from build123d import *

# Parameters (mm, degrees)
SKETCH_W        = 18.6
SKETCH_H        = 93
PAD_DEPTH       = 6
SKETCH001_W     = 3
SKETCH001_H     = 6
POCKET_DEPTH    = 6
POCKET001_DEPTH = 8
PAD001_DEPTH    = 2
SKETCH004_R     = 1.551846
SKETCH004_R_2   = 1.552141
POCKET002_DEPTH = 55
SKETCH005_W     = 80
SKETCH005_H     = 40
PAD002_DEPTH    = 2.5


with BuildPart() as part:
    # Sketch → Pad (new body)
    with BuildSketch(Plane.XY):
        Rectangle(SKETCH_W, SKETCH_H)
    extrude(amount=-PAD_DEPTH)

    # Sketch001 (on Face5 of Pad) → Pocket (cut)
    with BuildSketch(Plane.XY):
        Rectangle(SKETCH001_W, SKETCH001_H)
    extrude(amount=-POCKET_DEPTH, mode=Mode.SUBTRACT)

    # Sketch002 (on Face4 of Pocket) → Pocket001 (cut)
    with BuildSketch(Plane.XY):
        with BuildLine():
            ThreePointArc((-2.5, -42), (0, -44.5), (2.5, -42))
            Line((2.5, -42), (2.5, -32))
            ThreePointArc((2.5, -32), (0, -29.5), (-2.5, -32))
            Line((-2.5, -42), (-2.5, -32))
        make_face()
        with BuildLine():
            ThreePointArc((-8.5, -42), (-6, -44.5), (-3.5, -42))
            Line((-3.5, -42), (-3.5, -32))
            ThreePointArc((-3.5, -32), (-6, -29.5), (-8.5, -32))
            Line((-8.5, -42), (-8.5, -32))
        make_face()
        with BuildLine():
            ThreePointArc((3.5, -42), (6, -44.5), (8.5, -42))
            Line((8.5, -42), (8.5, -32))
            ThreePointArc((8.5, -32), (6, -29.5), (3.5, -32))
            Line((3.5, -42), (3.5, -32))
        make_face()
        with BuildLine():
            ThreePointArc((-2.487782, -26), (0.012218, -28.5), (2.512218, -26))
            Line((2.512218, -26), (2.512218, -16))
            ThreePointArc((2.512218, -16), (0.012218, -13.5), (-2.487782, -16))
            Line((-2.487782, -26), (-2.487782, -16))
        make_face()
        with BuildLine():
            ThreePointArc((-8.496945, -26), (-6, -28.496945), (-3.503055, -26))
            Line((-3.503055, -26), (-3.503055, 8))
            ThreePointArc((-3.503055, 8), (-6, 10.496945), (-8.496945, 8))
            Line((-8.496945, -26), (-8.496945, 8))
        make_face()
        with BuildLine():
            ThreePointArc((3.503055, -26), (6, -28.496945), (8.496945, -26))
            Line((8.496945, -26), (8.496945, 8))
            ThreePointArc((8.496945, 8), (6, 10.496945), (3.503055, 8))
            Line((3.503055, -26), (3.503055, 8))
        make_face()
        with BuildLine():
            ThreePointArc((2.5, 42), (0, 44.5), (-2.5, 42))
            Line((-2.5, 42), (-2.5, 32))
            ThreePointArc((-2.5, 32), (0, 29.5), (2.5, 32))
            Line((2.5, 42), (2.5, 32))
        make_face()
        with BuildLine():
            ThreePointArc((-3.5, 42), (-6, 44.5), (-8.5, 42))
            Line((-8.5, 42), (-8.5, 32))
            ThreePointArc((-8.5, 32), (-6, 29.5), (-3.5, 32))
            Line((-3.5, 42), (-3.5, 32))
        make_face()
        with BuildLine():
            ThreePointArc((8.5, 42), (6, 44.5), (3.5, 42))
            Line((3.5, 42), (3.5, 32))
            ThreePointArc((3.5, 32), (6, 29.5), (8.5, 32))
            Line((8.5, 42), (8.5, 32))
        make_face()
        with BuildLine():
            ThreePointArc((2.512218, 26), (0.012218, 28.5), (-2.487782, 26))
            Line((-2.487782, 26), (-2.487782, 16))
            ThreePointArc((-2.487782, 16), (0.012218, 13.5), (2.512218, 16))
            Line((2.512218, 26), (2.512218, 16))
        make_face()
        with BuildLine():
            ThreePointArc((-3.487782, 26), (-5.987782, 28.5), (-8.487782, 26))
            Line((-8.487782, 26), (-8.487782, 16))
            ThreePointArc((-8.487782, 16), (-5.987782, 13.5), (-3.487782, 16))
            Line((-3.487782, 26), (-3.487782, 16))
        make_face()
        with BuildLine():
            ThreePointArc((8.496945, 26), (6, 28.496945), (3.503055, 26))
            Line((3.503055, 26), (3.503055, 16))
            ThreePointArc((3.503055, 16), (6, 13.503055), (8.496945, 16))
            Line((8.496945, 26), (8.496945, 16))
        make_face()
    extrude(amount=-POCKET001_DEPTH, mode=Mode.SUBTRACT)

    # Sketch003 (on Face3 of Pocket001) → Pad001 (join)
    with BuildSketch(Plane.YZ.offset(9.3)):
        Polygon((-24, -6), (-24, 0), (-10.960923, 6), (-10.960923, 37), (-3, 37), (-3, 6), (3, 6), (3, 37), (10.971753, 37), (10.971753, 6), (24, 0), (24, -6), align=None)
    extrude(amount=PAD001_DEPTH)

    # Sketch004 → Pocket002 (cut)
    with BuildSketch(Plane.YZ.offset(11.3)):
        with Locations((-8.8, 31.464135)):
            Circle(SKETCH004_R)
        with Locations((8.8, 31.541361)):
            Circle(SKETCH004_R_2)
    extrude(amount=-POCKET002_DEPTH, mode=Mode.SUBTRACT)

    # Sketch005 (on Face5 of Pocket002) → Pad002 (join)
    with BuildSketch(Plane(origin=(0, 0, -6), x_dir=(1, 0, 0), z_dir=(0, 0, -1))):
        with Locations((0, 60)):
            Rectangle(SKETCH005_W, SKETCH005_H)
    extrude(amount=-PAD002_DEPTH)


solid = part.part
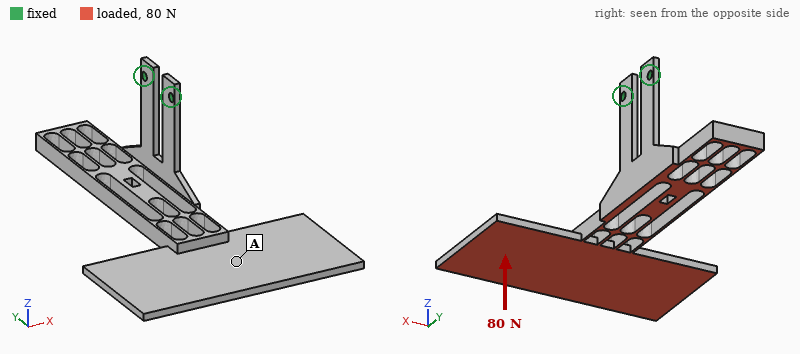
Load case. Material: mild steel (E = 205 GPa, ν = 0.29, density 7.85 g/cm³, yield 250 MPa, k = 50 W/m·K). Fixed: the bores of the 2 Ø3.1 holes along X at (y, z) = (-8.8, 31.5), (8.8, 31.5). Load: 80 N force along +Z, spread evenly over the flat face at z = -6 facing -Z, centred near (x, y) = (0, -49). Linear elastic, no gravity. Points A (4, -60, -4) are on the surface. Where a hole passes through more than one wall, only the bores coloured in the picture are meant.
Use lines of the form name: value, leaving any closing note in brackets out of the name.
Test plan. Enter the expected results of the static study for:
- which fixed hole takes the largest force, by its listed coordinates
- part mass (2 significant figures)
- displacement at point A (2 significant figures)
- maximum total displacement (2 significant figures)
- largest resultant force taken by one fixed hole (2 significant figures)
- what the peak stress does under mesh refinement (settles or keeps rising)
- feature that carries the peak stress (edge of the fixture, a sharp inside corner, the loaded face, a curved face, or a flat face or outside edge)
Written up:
which fixed hole takes the largest force, by its listed coordinates: (-8.8, 31.5)
part mass: 110 g
displacement at point A: 0.36 mm
maximum total displacement: 1.2 mm
largest resultant force taken by one fixed hole: 280 N
what the peak stress does under mesh refinement: keeps rising
feature that carries the peak stress: a sharp inside corner
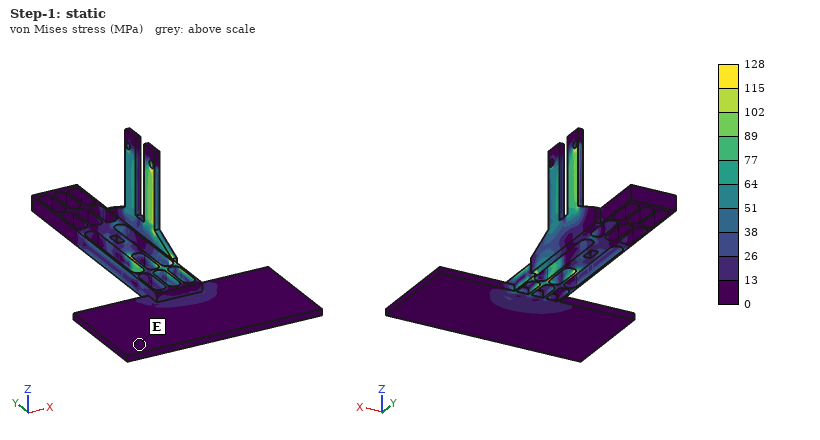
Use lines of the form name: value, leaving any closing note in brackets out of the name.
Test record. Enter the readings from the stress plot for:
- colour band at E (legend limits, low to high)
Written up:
colour band at E: 0 to 13 MPa
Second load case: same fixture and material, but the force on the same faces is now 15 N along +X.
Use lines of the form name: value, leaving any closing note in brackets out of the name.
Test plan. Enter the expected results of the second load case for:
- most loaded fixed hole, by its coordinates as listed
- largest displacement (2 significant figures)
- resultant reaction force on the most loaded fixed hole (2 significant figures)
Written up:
most loaded fixed hole, by its coordinates as listed: (-8.8, 31.5)
largest displacement: 0.65 mm
resultant reaction force on the most loaded fixed hole: 23 N
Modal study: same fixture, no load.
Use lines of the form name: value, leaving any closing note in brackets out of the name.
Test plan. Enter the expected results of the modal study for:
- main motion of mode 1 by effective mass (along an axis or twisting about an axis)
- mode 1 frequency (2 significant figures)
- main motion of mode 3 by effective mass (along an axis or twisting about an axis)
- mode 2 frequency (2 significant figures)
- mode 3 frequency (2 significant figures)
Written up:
main motion of mode 1 by effective mass: along X
mode 1 frequency: 98 Hz
main motion of mode 3 by effective mass: along Z
mode 2 frequency: 160 Hz
mode 3 frequency: 370 Hz
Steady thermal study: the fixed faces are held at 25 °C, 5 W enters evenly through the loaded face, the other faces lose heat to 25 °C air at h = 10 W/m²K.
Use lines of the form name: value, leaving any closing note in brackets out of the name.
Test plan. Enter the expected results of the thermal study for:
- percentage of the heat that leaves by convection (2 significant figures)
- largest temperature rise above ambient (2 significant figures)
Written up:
percentage of the heat that leaves by convection: 80 %
largest temperature rise above ambient: 64 K
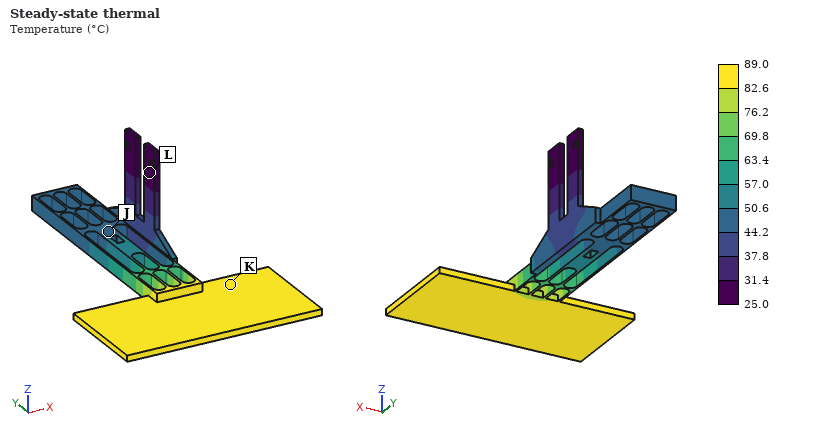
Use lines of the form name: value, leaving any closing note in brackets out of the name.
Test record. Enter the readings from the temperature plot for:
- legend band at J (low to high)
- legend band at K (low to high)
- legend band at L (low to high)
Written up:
legend band at J: 44.2 to 50.6 °C
legend band at K: 82.6 to 89.0 °C
legend band at L: 25.0 to 31.4 °C
